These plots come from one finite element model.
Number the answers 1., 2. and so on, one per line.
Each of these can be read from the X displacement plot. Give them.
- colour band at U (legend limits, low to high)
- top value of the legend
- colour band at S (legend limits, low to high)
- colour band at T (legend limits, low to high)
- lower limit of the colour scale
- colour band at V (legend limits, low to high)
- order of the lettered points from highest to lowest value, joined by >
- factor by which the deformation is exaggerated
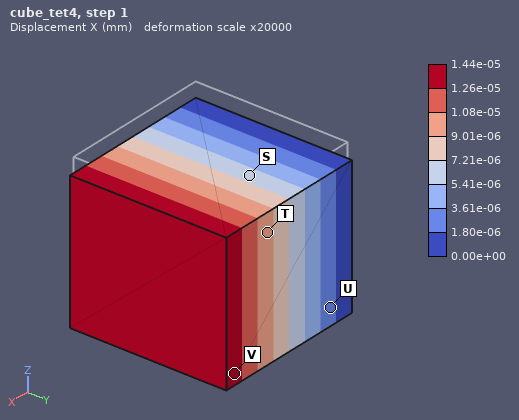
1. 1.80e-06 to 3.61e-06 mm
2. 1.44e-05 mm
3. 5.41e-06 to 7.21e-06 mm
4. 9.01e-06 to 1.08e-05 mm
5. 0.00e+00 mm
6. 1.26e-05 to 1.44e-05 mm
7. V > T > S > U
8. 20000
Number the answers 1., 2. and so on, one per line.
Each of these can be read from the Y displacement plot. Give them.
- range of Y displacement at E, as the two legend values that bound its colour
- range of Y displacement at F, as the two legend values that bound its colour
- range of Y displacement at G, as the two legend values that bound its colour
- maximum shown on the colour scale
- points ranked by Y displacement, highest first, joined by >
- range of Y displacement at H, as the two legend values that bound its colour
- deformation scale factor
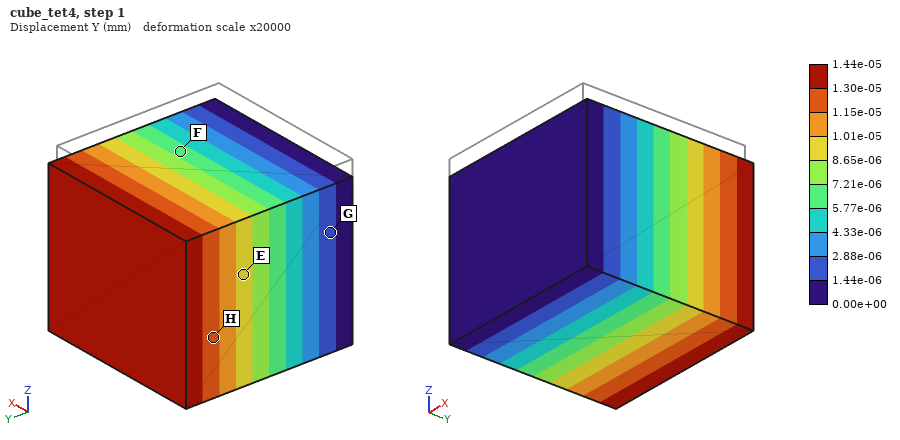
1. 8.65e-06 to 1.01e-05 mm
2. 5.77e-06 to 7.21e-06 mm
3. 1.44e-06 to 2.88e-06 mm
4. 1.44e-05 mm
5. H > E > F > G
6. 1.15e-05 to 1.30e-05 mm
7. 20000
